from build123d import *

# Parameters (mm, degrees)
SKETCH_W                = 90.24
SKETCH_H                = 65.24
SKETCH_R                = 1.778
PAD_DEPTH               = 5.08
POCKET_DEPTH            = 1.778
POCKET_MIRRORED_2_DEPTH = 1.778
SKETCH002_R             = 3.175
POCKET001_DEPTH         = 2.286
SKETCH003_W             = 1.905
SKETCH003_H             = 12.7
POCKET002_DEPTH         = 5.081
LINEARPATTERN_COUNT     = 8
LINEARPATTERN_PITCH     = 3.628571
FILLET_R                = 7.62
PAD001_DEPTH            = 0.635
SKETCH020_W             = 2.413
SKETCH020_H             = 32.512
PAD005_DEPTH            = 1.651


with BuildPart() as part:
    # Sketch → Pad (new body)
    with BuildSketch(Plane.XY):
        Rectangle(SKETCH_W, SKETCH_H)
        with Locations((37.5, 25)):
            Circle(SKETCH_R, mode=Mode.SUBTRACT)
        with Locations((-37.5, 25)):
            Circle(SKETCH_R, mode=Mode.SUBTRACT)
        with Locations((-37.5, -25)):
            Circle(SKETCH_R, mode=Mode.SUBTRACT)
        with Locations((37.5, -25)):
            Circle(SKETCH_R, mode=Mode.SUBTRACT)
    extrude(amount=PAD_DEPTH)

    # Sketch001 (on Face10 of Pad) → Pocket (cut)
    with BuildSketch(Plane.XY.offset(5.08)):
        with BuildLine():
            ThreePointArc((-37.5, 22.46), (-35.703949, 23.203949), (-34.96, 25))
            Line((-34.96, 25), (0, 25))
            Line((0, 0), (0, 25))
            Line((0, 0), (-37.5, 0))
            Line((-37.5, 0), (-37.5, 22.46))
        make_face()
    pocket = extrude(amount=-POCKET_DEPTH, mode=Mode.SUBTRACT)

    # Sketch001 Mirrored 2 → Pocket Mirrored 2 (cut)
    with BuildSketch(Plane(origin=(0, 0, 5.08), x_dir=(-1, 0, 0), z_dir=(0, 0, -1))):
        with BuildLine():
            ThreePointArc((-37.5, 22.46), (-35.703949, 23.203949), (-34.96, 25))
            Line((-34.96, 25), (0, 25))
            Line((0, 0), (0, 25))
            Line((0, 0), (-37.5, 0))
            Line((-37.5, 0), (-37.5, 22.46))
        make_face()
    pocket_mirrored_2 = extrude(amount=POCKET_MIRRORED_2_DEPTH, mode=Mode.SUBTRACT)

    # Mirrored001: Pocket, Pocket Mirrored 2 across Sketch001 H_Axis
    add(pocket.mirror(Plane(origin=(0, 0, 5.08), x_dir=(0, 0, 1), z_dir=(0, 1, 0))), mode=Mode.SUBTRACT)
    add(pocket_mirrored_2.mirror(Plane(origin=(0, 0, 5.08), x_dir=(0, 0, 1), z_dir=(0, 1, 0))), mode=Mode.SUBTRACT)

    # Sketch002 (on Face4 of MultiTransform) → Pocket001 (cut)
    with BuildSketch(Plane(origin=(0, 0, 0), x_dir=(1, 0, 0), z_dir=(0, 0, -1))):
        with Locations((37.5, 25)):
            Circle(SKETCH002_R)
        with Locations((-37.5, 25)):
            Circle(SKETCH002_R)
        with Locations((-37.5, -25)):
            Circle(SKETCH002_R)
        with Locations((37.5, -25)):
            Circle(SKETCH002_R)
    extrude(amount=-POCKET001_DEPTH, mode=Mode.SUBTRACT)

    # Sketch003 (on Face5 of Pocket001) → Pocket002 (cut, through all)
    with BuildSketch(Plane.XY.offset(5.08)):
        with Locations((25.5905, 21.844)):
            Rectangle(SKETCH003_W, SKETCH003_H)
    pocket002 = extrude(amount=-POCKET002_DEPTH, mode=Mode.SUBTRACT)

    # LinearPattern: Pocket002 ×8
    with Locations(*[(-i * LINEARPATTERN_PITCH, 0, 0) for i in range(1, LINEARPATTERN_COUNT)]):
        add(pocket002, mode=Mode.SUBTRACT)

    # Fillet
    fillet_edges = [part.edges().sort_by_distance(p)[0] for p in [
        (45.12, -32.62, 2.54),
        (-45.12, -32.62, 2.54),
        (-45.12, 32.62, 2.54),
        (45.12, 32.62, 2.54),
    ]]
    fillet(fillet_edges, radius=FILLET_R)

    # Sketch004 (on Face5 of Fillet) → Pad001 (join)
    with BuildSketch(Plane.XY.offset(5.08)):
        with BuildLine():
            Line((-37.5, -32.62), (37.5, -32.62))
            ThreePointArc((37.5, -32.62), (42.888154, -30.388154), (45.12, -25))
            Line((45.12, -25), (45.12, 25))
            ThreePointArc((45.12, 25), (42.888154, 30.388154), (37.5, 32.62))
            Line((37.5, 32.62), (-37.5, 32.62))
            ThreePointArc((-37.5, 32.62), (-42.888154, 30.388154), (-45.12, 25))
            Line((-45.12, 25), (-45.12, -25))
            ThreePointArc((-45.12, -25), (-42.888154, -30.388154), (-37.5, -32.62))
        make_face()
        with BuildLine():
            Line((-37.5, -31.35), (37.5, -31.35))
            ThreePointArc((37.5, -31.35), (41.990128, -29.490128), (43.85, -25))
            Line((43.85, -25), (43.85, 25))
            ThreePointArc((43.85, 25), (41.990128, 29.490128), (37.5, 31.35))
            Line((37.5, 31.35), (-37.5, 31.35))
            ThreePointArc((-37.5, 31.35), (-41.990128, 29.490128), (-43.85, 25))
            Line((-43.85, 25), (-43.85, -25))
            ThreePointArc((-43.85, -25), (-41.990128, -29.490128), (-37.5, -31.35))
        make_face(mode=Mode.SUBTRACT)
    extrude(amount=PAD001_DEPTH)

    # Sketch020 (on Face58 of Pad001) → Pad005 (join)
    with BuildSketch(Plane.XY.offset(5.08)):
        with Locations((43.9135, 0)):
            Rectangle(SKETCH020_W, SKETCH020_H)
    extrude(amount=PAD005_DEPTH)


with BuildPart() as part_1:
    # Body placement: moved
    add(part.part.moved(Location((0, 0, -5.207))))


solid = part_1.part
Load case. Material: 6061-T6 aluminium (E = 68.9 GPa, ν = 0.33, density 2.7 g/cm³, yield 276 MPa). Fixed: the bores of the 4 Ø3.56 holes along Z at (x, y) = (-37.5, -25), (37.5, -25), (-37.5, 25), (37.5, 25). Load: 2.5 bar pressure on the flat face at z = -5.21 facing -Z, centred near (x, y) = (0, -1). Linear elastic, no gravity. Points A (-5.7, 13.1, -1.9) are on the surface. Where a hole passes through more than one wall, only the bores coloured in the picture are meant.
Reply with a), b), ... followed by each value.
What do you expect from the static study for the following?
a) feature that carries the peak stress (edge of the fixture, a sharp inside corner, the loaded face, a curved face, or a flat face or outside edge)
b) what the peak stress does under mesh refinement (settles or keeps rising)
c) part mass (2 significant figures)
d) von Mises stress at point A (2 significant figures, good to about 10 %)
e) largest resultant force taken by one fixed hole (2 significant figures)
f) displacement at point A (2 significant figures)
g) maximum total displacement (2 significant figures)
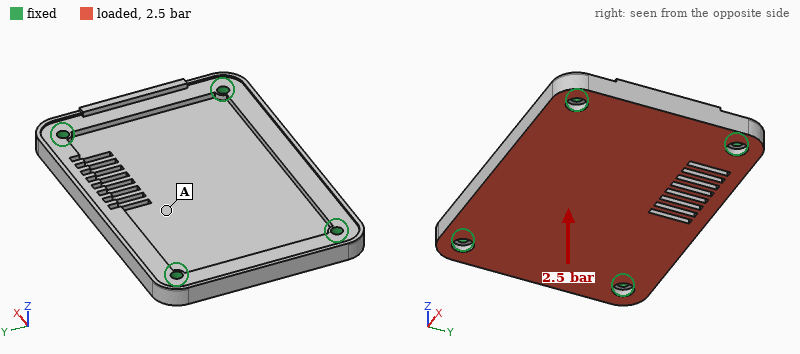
a) edge of the fixture
b) keeps rising
c) 60 g
d) 19 MPa
e) 720 N
f) 0.11 mm
g) 0.12 mm
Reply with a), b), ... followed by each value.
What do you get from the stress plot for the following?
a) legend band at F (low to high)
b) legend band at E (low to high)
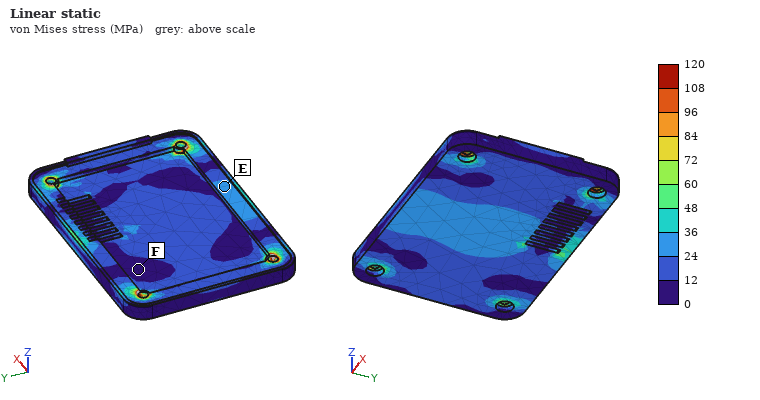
a) 0 to 12 MPa
b) 24 to 36 MPa
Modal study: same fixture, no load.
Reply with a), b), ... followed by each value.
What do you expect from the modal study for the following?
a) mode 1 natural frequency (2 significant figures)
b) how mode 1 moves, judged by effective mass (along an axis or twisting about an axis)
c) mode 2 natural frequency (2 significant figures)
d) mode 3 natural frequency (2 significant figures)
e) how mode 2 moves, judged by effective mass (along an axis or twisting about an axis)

a) 2800 Hz
b) along Z
c) 4100 Hz
d) 6000 Hz
e) twisting about X
